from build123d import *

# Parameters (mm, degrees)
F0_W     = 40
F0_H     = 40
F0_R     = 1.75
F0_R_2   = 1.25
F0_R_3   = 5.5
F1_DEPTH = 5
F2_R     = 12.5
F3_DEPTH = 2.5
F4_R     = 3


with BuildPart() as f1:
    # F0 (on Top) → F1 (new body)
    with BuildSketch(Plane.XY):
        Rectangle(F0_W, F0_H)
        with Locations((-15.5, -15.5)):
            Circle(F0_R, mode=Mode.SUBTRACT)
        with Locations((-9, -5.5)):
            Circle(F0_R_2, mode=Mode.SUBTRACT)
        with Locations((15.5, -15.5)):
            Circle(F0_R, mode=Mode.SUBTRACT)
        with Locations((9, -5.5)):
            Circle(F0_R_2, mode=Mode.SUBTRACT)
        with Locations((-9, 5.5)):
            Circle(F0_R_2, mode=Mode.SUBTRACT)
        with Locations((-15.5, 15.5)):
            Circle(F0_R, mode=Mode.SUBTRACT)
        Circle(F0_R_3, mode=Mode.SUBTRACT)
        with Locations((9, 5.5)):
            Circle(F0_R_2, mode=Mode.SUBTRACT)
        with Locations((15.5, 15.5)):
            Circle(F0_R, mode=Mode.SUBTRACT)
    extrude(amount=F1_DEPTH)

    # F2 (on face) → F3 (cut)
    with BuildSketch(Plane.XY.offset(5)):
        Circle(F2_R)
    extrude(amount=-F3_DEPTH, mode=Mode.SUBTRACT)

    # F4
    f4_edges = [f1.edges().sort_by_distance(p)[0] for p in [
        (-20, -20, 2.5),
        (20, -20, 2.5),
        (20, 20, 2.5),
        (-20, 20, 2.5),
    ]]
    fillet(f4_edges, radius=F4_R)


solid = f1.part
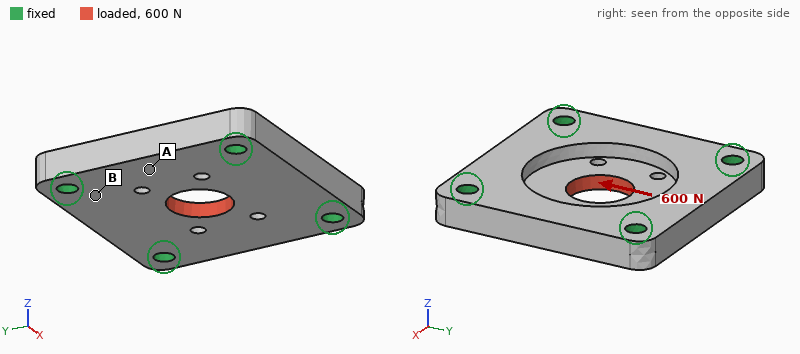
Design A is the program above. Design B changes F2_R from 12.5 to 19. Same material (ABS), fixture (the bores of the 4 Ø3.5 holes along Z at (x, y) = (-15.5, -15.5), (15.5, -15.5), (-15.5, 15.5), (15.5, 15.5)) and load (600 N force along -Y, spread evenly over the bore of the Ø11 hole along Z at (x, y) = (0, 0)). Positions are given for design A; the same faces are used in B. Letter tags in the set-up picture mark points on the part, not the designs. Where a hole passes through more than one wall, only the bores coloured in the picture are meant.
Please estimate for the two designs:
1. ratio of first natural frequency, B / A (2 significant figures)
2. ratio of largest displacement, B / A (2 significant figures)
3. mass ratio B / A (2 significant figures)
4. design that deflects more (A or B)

0.66
1.1
0.74
B
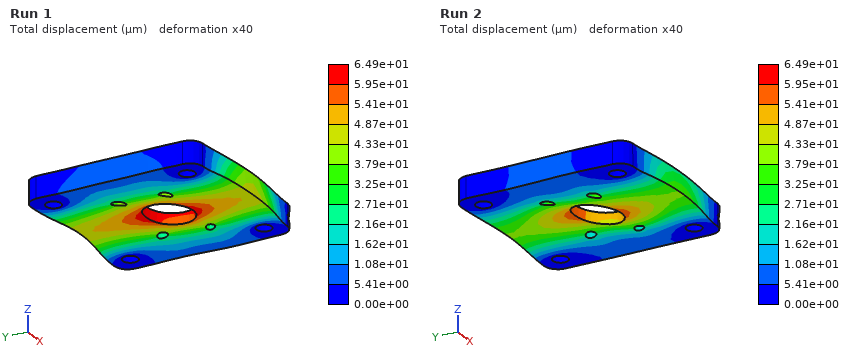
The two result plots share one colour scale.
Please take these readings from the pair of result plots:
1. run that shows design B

Run 1
